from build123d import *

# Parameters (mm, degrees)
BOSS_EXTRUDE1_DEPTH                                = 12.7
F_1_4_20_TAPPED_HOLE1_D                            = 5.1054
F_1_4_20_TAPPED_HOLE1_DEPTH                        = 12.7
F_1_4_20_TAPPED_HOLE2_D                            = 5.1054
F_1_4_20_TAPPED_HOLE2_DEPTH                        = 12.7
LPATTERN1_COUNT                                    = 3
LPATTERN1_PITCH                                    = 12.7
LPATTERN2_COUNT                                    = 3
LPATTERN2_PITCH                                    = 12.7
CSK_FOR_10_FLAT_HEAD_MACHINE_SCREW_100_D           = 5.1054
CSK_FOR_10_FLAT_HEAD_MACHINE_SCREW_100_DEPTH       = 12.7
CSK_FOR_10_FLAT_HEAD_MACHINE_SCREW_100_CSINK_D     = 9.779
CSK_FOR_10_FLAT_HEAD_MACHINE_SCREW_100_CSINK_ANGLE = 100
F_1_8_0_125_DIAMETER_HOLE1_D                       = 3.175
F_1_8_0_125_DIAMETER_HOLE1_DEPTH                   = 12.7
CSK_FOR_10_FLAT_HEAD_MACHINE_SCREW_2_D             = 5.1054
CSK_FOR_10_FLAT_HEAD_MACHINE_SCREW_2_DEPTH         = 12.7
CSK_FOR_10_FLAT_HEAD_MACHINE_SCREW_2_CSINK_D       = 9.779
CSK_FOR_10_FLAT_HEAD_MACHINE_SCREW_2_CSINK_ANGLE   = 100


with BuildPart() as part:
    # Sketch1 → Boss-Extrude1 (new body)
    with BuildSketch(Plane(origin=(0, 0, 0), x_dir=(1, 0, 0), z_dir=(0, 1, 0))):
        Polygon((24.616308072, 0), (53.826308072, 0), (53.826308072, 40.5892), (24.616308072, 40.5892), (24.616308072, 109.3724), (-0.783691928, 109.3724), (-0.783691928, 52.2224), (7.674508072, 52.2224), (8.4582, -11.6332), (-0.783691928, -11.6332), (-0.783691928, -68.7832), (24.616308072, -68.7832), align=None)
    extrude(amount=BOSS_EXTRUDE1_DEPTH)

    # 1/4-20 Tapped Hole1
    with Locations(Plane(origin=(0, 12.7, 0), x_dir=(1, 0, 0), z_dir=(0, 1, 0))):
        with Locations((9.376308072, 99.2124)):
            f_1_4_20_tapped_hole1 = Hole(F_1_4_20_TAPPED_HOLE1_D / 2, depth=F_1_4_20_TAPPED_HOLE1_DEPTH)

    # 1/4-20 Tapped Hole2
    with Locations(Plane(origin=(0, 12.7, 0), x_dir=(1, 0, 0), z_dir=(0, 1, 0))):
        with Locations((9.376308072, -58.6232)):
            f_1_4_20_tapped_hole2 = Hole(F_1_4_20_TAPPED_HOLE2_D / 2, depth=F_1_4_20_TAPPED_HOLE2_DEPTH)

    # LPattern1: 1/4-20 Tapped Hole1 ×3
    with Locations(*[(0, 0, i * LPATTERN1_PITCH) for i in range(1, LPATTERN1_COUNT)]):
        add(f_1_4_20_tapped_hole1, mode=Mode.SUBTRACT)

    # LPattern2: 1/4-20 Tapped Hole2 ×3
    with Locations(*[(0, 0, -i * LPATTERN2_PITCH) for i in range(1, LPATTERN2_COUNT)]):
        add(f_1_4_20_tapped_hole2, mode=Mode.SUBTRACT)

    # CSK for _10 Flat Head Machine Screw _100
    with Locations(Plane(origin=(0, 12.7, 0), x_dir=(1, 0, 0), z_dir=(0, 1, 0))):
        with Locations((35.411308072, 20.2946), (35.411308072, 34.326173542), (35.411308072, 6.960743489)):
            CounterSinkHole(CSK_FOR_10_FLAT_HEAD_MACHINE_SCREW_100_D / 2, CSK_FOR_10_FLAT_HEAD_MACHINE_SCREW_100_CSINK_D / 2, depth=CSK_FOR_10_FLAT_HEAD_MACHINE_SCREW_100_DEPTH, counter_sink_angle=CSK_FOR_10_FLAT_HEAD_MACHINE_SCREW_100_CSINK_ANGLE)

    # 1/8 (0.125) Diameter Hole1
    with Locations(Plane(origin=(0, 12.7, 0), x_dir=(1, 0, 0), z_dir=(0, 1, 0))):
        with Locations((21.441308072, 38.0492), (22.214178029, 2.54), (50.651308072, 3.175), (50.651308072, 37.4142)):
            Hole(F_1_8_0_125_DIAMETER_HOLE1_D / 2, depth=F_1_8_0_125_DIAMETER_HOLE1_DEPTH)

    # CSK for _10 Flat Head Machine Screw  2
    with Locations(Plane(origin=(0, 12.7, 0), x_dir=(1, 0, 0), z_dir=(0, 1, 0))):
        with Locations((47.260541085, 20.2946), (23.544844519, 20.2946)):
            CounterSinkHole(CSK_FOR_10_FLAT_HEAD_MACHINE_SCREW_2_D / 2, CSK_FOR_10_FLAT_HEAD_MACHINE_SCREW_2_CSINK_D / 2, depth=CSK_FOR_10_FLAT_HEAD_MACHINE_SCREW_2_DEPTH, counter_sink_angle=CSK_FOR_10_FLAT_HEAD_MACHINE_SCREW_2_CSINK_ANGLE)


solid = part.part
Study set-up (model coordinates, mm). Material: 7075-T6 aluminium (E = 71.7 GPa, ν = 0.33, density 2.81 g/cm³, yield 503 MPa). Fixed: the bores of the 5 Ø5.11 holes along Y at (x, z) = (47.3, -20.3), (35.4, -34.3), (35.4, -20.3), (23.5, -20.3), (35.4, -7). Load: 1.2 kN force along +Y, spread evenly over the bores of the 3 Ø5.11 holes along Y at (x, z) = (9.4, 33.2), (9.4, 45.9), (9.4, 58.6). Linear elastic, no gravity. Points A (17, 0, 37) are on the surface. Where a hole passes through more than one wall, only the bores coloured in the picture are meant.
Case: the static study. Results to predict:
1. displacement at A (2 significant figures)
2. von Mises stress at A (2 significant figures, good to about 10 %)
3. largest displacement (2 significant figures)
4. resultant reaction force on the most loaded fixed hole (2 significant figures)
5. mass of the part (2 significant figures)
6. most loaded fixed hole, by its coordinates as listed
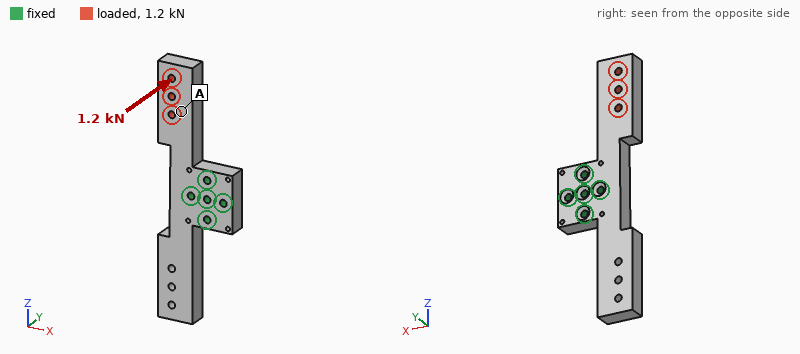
0.36 mm
22 MPa
0.74 mm
2.3 kN
170 g
(35.4, -7)
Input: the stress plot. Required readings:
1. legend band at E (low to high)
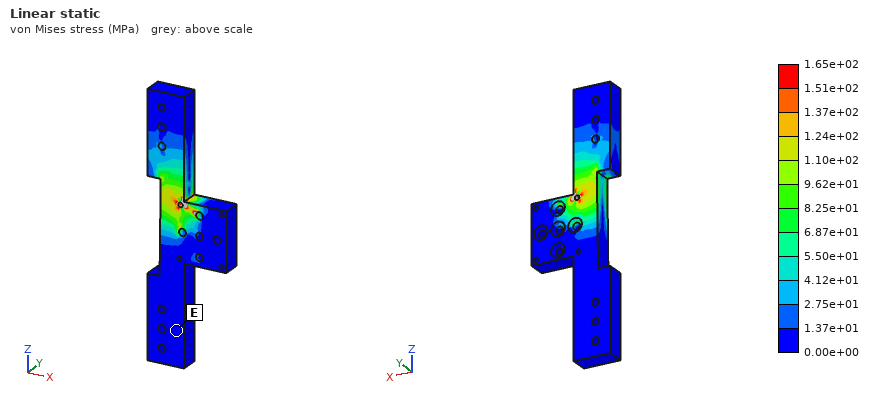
0.00e+00 to 1.37e+01 MPa
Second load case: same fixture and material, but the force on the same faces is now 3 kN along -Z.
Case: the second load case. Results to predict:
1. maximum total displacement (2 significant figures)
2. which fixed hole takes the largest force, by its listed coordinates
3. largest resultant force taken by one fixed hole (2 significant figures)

0.15 mm
(23.5, -20.3)
3.2 kN
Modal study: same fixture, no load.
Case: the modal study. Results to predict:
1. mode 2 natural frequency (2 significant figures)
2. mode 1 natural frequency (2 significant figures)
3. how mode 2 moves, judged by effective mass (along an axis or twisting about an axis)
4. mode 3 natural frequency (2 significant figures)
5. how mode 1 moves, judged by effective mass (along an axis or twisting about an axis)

1300 Hz
1200 Hz
along Y
1800 Hz
twisting about X
